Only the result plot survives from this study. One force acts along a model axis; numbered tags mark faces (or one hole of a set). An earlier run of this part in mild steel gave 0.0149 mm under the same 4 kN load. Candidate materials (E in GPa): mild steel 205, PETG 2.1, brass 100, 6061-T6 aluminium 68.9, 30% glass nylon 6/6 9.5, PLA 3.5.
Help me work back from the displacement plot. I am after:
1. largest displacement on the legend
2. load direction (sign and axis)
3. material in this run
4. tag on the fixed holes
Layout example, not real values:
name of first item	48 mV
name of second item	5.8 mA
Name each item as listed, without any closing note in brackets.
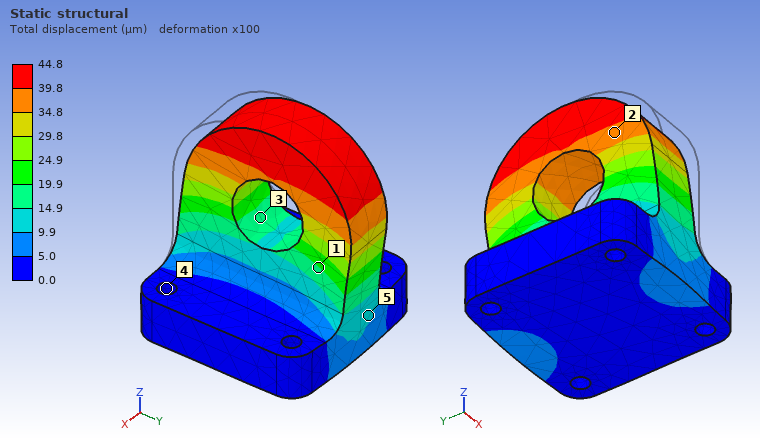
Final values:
largest displacement on the legend	44.8 µm
load direction	+Y
material in this run	6061-T6 aluminium
tag on the fixed holes	4
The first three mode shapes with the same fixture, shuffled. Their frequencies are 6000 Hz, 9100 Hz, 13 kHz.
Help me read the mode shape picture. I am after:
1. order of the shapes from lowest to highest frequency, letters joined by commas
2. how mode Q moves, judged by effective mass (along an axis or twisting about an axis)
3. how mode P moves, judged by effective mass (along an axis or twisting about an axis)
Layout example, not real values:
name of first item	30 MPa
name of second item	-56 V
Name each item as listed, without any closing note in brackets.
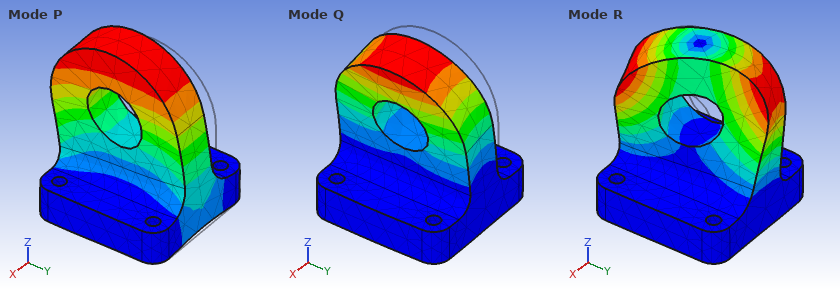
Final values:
order of the shapes from lowest to highest frequency, letters joined by commas	Q, P, R
how mode Q moves, judged by effective mass	along X
how mode P moves, judged by effective mass	along Y
